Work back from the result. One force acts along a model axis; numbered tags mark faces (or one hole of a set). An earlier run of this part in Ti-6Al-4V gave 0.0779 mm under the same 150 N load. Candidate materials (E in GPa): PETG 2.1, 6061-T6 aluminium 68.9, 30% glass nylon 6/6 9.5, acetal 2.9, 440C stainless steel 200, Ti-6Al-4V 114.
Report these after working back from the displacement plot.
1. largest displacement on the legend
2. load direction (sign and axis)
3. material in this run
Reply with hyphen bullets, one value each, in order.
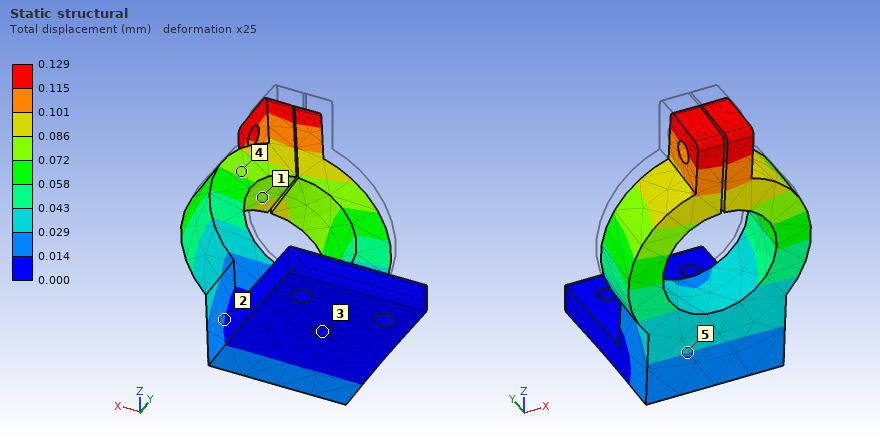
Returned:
- 0.129 mm
- -Y
- 6061-T6 aluminium
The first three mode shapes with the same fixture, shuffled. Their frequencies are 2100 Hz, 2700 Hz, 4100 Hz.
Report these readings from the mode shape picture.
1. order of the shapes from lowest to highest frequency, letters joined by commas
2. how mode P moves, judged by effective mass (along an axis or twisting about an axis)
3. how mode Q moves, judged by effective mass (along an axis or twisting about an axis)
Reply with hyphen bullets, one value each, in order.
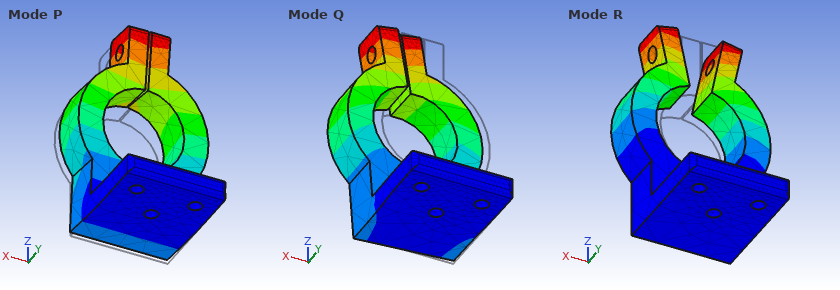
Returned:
- P, Q, R
- along Y
- along X
